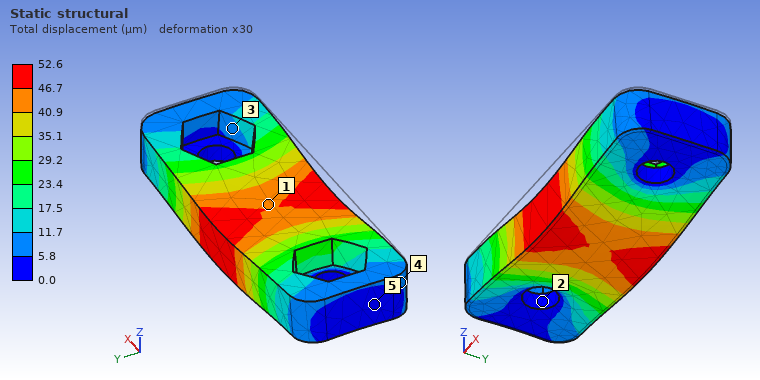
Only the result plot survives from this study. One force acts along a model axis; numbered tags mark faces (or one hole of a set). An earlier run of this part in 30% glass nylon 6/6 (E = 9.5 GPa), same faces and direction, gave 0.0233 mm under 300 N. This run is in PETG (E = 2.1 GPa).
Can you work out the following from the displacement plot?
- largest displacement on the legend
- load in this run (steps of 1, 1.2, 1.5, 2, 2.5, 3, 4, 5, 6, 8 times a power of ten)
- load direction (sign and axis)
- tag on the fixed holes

52.6 µm
150 N
-Z
2
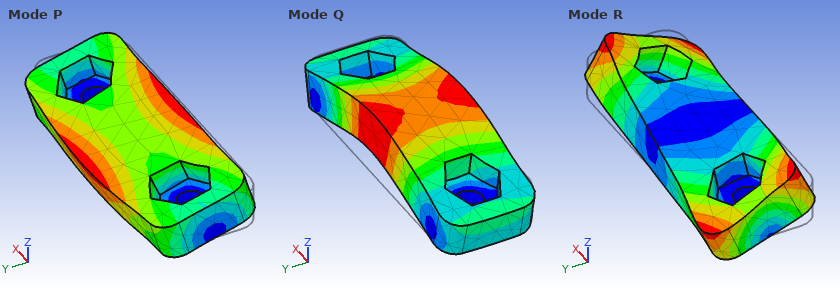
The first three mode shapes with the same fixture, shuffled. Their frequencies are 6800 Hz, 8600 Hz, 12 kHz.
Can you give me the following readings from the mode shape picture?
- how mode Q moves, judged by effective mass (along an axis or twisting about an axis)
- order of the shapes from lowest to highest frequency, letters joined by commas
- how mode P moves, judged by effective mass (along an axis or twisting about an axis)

along Z
P, Q, R
along Y
